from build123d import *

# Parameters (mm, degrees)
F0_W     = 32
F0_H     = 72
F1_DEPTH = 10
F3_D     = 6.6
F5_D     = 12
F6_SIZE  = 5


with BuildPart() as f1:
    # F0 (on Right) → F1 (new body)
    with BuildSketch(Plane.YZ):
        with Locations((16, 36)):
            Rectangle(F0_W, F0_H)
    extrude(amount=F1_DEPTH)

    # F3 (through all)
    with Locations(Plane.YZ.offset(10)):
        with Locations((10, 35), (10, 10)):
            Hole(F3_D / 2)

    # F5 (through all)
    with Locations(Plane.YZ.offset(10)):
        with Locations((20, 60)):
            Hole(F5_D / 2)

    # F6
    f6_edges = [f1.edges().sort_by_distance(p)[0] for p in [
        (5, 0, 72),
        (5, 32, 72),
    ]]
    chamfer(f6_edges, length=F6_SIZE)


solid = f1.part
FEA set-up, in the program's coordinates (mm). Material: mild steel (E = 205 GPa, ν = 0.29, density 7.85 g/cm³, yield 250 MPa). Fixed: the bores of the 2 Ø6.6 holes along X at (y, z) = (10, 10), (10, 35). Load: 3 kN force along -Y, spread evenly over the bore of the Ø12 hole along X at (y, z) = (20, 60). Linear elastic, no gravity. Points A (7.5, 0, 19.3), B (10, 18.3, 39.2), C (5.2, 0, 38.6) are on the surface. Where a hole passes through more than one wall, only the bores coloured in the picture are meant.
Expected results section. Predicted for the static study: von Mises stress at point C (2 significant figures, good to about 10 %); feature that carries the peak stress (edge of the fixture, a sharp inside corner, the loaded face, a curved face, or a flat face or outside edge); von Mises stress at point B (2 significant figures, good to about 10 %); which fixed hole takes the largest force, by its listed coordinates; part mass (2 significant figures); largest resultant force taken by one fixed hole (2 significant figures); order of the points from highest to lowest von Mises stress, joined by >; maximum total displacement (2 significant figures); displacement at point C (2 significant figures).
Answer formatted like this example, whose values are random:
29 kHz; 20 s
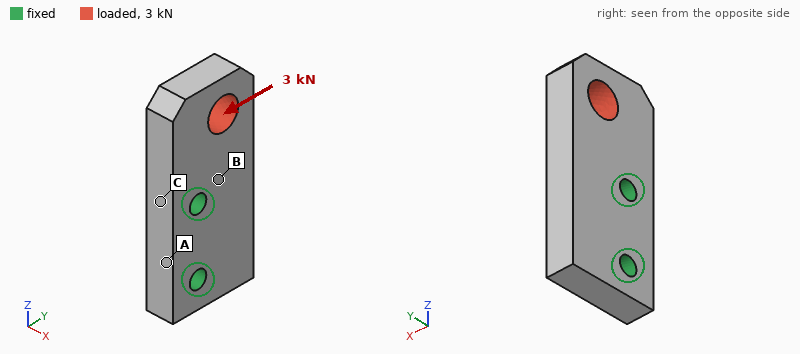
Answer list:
46 MPa; edge of the fixture; 24 MPa; (10, 35); 160 g; 5.1 kN; C > B > A; 18 µm; 2.8 µm
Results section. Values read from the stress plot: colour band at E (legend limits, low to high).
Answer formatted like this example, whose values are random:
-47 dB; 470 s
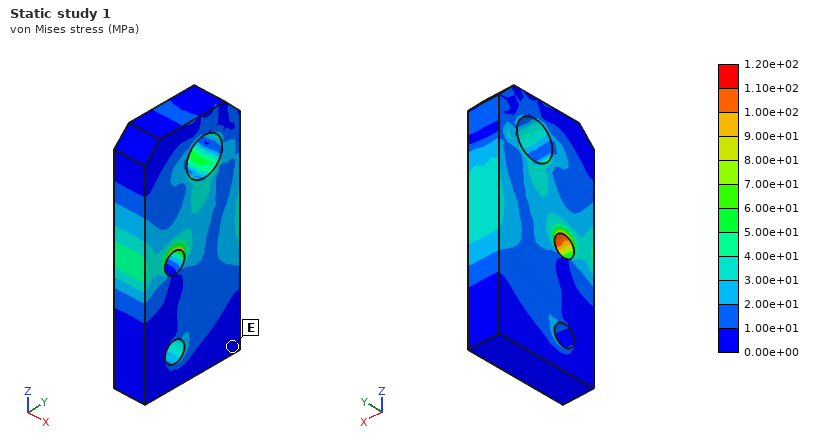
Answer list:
0.00e+00 to 1.00e+01 MPa
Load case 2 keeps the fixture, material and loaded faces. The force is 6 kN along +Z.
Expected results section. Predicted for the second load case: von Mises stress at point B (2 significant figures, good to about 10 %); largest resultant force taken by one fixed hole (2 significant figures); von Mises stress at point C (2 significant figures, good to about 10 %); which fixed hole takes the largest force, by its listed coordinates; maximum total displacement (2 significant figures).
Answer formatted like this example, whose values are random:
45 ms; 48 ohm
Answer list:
21 MPa; 4.6 kN; 11 MPa; (10, 35); 11 µm
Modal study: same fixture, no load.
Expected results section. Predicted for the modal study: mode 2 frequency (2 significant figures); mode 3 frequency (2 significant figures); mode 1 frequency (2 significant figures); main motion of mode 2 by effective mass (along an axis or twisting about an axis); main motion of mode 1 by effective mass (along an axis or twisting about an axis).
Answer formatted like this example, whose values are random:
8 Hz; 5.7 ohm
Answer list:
10 kHz; 11 kHz; 5900 Hz; along Y; along X
